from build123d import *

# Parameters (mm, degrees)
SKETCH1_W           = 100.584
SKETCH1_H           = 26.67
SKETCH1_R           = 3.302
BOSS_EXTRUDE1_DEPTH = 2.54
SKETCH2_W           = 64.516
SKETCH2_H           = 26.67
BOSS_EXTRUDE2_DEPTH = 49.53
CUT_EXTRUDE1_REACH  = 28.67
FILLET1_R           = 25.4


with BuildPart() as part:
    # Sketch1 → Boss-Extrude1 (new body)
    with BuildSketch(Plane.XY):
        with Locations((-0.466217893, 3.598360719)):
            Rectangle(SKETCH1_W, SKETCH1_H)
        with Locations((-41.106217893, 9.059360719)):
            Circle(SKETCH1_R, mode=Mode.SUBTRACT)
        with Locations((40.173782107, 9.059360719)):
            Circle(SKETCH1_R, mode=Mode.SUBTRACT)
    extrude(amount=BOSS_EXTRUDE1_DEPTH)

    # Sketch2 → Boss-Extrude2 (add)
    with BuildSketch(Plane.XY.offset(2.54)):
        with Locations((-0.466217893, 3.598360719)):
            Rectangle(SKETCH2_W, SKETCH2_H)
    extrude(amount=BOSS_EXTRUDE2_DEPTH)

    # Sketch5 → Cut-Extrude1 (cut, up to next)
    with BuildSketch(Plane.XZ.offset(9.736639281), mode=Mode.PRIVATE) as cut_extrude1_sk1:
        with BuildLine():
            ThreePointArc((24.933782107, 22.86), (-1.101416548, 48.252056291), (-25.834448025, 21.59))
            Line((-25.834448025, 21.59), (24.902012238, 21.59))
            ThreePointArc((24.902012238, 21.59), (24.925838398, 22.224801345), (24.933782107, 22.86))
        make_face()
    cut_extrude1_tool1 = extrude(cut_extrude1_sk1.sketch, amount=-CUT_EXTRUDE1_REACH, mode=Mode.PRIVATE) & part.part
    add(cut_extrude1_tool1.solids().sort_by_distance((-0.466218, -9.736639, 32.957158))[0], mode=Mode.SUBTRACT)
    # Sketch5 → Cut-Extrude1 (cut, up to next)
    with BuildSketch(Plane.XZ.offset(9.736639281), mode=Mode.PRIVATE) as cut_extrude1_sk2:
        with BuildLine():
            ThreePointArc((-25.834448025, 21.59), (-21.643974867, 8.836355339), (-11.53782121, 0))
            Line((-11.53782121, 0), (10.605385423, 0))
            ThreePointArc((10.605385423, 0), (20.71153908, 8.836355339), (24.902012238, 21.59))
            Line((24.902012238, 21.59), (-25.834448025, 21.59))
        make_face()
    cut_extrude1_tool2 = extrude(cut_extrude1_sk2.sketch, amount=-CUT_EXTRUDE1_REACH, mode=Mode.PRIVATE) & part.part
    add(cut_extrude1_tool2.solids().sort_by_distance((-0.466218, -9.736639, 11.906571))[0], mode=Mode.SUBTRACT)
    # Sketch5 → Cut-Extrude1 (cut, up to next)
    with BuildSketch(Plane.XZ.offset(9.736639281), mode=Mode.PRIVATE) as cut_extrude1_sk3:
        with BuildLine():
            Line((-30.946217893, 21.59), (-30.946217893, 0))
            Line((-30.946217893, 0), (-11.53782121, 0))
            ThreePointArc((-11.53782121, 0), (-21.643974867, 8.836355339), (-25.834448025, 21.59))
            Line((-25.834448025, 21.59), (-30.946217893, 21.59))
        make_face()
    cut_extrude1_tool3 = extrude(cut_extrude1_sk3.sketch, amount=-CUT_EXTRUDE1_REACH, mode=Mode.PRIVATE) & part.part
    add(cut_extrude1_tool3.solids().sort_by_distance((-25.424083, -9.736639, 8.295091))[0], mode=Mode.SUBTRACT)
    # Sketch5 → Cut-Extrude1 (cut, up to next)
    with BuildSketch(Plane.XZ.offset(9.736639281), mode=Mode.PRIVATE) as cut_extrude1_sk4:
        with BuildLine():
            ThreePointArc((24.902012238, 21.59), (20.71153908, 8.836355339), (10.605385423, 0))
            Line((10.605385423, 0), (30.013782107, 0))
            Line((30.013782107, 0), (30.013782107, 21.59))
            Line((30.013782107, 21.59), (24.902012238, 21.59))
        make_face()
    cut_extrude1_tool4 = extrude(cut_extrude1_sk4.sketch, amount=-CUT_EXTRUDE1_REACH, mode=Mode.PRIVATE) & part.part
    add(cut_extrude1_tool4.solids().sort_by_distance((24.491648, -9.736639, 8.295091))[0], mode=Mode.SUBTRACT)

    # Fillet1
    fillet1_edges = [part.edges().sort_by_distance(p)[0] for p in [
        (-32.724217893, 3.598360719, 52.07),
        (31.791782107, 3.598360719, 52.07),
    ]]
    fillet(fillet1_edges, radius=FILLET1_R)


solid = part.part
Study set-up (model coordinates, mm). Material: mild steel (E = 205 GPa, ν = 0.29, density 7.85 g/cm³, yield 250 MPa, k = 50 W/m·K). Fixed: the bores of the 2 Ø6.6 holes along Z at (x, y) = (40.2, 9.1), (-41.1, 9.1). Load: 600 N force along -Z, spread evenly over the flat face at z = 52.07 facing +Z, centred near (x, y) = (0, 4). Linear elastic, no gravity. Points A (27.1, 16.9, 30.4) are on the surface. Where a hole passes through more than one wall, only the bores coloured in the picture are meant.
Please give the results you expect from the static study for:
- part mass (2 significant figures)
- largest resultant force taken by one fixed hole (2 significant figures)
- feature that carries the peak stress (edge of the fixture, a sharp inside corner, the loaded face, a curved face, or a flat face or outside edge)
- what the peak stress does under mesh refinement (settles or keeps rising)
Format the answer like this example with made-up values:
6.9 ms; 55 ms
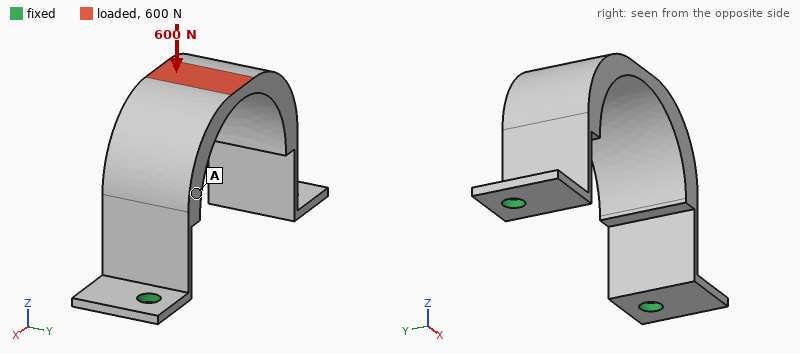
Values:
160 g; 320 N; edge of the fixture; keeps rising
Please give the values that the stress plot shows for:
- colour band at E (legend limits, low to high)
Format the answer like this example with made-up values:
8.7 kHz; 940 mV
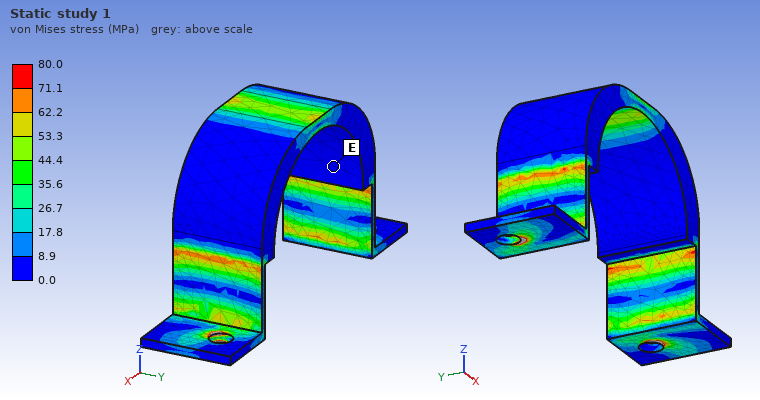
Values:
0.0 to 8.9 MPa
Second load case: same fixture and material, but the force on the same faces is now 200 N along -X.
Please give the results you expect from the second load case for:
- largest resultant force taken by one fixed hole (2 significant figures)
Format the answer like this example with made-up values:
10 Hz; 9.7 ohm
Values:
160 N
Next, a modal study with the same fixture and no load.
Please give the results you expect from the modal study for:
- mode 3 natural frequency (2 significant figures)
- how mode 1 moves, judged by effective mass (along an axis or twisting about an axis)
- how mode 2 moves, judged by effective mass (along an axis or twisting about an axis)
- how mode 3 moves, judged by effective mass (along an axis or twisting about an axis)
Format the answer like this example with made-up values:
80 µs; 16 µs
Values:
1900 Hz; along Y; along X; twisting about Z
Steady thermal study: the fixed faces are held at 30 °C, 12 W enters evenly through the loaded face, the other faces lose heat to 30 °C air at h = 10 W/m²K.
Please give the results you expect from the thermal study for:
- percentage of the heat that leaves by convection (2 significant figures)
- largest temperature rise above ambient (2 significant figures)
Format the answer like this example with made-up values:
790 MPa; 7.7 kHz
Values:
36 %; 74 K
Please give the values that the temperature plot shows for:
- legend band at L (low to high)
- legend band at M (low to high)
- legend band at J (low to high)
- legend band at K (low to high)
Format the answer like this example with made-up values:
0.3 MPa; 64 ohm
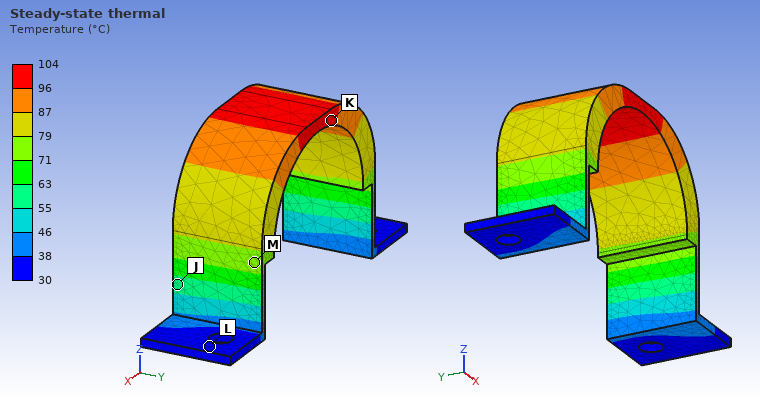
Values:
30 to 38 °C; 71 to 79 °C; 55 to 63 °C; 96 to 104 °C
